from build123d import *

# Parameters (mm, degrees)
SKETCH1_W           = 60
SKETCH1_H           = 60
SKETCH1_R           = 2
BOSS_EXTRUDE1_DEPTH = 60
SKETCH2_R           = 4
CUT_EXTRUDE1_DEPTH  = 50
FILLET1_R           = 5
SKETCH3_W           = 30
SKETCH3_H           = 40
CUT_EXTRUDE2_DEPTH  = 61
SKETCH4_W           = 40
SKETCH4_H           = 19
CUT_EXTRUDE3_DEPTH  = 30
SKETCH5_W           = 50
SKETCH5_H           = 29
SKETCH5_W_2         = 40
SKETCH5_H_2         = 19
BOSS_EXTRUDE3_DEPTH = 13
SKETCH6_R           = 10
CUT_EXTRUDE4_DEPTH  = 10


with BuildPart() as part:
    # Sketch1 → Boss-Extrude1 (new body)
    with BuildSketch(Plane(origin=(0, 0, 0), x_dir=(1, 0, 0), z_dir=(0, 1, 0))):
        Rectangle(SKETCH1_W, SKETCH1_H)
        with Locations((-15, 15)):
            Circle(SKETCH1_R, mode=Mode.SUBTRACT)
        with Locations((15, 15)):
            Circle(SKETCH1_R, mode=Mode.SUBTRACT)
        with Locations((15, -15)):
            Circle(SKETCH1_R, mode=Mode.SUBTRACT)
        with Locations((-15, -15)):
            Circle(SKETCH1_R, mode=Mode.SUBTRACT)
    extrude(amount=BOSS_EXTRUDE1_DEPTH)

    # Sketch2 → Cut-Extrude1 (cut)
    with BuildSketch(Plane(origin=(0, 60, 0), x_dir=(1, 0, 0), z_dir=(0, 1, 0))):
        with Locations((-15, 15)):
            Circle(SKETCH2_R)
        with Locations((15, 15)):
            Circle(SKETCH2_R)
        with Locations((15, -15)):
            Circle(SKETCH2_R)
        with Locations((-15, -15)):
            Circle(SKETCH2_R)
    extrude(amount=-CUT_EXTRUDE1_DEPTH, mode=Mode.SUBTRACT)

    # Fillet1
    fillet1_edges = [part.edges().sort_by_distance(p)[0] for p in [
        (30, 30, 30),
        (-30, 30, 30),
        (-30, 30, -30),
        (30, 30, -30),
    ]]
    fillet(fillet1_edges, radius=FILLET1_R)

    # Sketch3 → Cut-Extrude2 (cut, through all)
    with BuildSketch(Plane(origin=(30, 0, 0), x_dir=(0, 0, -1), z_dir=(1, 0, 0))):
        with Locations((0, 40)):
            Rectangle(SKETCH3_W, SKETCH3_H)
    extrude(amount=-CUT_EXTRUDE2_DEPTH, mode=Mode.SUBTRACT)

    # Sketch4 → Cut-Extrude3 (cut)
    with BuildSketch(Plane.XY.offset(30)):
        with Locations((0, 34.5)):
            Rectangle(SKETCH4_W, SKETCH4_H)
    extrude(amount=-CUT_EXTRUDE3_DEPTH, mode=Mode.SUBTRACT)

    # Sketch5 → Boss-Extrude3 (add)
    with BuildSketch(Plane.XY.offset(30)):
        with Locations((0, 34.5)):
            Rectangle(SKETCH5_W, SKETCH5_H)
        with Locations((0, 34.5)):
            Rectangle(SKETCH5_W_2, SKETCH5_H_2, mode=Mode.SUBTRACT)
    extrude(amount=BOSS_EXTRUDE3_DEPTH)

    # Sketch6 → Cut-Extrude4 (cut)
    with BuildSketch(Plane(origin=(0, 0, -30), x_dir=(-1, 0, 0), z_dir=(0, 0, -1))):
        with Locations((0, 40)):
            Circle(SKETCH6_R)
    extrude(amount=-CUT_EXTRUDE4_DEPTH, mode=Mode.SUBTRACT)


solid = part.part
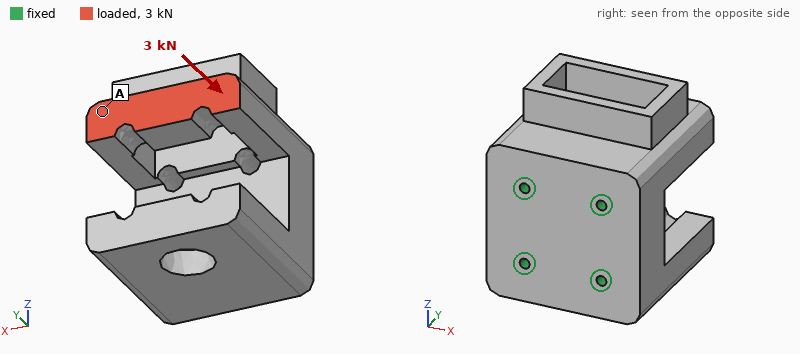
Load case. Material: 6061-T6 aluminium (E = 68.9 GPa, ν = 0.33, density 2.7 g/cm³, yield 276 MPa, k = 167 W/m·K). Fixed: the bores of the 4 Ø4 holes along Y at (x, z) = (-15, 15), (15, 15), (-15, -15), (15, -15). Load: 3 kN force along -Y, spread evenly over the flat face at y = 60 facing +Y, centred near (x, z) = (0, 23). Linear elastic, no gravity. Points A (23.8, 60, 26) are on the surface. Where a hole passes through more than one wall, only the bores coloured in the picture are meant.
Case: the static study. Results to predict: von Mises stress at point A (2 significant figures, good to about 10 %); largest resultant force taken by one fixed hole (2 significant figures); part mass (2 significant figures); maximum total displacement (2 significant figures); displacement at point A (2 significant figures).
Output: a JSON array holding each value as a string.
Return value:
["3.6 MPa", "1.8 kN", "360 g", "20 µm", "12 µm"]
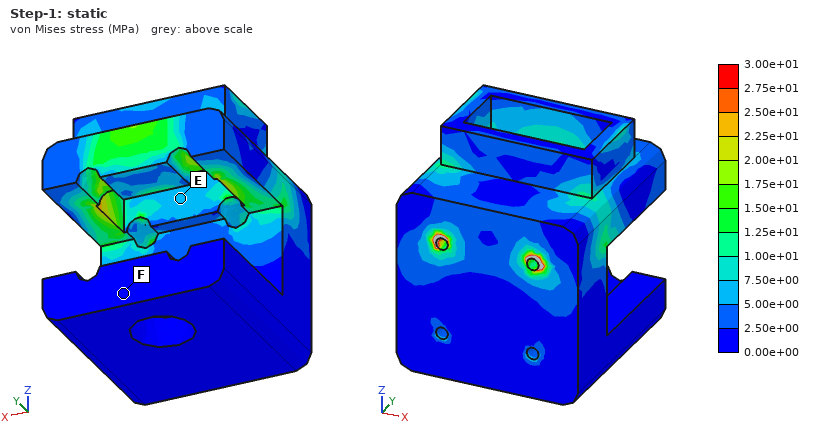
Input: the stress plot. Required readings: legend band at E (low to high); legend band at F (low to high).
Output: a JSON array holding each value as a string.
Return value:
["5.00e+00 to 7.50e+00 MPa", "0.00e+00 to 2.50e+00 MPa"]
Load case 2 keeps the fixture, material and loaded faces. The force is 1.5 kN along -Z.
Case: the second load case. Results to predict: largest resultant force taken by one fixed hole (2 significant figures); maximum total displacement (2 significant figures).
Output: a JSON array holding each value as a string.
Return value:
["1.5 kN", "0.11 mm"]
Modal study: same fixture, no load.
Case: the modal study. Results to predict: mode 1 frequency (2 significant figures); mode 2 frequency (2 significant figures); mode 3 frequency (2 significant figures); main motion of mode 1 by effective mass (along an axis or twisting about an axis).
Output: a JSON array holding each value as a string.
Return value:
["3200 Hz", "4100 Hz", "4200 Hz", "along Z"]
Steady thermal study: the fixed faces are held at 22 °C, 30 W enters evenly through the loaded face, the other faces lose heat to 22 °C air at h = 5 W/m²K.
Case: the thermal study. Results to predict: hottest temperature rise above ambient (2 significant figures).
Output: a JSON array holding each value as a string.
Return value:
["22 K"]
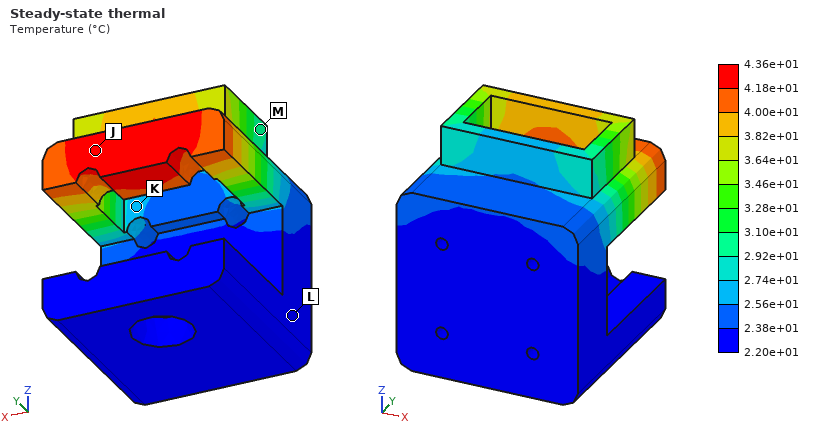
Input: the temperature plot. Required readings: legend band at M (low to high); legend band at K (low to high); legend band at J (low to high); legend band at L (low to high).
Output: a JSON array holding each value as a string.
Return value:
["2.92e+01 to 3.10e+01 °C", "2.56e+01 to 2.74e+01 °C", "4.18e+01 to 4.36e+01 °C", "2.20e+01 to 2.38e+01 °C"]
